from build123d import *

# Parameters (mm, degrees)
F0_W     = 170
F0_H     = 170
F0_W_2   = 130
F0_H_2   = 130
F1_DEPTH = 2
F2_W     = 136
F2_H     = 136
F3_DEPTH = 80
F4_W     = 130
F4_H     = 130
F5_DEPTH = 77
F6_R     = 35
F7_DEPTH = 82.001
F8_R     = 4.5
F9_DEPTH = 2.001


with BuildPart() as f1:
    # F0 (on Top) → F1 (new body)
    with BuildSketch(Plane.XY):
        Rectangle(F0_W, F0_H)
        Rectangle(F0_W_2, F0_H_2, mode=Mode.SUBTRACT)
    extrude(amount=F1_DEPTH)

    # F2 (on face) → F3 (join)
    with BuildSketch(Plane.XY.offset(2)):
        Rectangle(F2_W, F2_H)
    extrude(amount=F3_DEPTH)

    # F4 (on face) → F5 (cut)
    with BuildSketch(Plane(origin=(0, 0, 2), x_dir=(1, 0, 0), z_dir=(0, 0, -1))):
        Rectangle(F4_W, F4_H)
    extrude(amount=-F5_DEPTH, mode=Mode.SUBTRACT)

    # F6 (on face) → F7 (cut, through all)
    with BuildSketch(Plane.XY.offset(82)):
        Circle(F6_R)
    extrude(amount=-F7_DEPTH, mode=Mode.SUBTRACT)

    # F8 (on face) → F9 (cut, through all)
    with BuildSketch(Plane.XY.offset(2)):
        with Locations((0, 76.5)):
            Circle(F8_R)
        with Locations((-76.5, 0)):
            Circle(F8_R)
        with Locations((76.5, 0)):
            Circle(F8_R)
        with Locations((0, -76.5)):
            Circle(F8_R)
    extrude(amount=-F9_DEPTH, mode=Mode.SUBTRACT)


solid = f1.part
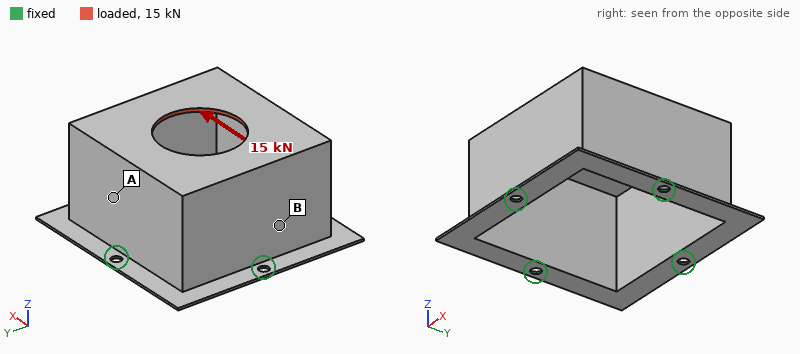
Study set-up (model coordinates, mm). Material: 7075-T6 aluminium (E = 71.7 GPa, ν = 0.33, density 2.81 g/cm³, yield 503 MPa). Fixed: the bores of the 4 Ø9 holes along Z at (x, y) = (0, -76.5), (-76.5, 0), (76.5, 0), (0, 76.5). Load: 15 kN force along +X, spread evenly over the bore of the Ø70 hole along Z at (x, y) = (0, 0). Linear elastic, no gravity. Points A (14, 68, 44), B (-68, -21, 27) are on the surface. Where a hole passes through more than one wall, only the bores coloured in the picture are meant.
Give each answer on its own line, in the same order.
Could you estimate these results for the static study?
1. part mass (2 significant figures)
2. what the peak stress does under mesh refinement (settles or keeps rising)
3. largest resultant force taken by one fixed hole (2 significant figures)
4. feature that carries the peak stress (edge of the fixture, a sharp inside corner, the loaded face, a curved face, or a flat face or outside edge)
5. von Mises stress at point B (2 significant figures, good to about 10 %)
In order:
530 g
keeps rising
8.7 kN
edge of the fixture
92 MPa
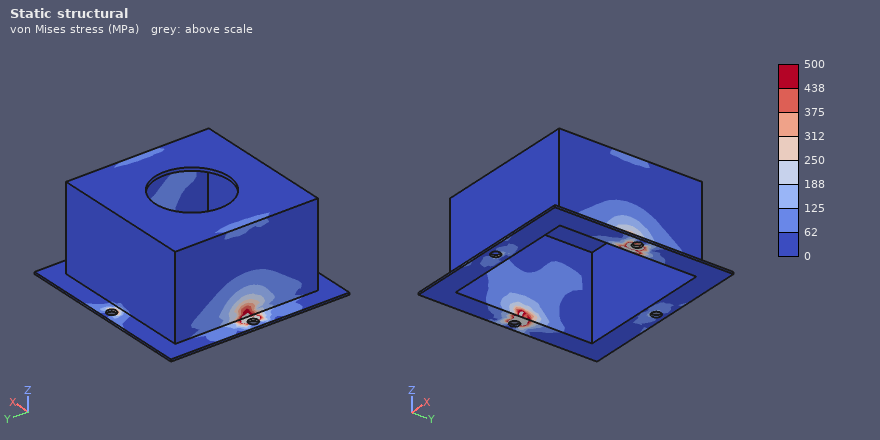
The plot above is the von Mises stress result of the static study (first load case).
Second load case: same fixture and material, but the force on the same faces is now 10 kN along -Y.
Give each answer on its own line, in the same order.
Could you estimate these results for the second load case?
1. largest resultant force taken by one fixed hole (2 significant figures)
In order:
5.8 kN
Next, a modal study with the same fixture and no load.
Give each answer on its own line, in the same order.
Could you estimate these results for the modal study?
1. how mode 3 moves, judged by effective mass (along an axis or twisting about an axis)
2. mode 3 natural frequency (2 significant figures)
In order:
along Z
1500 Hz
